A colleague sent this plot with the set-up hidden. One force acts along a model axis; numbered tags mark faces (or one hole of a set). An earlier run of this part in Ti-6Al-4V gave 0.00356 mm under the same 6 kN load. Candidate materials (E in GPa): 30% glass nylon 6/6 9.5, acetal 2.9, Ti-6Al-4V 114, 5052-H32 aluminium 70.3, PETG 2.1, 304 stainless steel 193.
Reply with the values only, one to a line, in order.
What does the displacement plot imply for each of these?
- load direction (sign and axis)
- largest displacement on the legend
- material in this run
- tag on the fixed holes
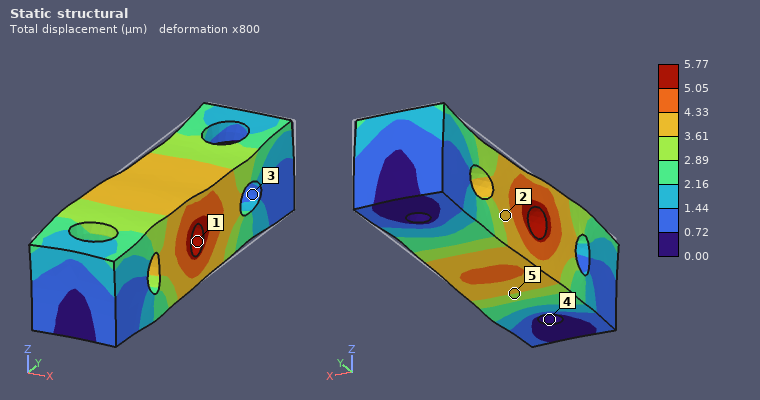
-Y
5.77 µm
5052-H32 aluminium
4
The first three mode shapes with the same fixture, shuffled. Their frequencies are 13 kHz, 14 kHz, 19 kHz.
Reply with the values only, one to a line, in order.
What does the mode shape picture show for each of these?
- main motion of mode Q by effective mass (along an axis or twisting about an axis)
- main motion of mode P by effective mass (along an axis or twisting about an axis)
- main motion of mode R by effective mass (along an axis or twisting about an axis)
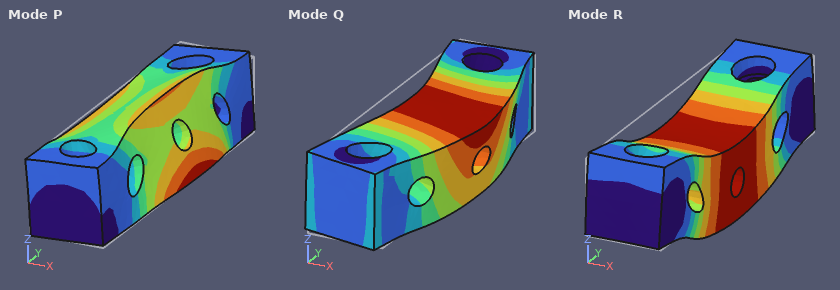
along X
twisting about Y
along Z
